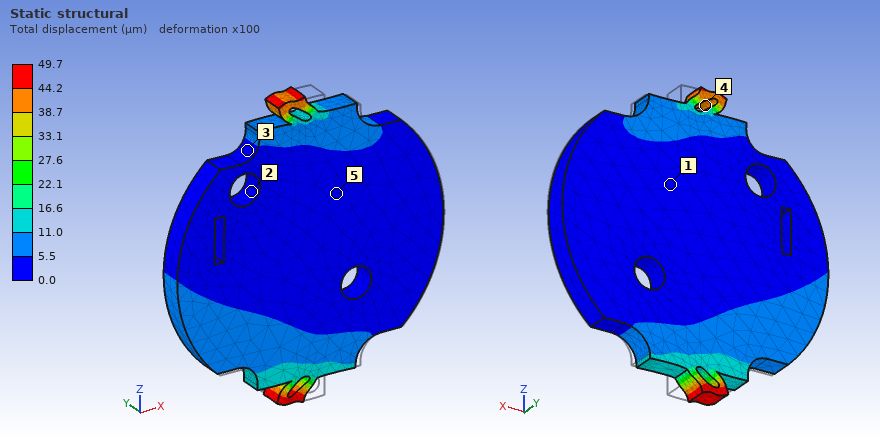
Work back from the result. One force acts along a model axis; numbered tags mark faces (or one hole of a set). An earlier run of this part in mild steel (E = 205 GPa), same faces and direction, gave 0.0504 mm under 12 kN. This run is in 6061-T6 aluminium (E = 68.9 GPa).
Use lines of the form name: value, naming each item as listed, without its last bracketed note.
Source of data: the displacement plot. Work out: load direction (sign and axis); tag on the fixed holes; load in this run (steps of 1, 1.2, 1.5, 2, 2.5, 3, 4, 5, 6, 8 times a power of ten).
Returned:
load direction: -X
tag on the fixed holes: 2
load in this run: 4 kN
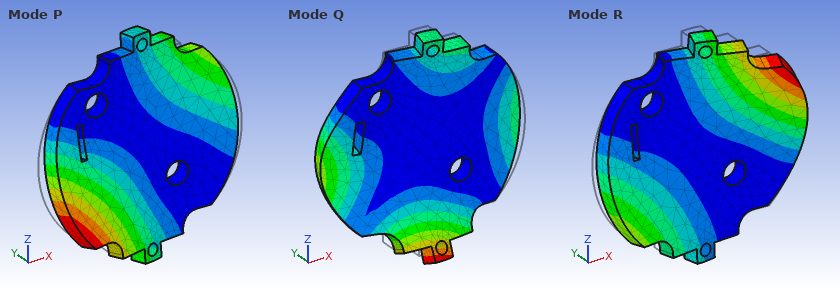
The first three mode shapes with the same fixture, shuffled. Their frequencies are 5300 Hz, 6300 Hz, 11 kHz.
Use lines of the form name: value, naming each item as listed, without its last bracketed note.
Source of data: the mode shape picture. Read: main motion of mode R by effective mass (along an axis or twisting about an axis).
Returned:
main motion of mode R by effective mass: along Y
